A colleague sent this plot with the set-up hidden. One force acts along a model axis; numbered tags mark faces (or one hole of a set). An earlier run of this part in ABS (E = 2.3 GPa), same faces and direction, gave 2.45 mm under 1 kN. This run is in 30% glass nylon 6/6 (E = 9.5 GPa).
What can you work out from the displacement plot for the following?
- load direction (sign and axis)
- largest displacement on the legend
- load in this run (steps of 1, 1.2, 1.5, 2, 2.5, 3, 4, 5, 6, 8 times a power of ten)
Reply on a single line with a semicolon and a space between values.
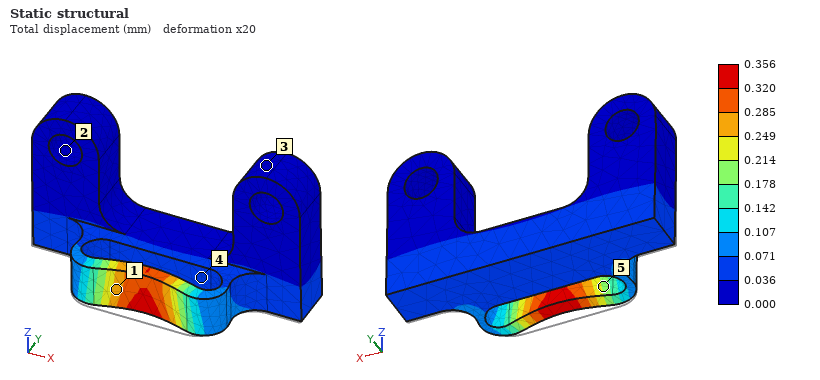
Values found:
+Y; 0.356 mm; 600 N
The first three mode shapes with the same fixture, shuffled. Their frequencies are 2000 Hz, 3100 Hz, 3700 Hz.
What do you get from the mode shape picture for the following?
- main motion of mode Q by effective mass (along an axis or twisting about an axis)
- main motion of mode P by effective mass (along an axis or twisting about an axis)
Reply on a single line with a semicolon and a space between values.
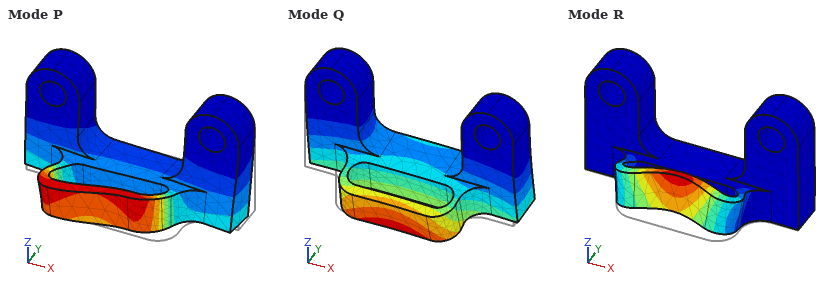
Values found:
along Y; along X
